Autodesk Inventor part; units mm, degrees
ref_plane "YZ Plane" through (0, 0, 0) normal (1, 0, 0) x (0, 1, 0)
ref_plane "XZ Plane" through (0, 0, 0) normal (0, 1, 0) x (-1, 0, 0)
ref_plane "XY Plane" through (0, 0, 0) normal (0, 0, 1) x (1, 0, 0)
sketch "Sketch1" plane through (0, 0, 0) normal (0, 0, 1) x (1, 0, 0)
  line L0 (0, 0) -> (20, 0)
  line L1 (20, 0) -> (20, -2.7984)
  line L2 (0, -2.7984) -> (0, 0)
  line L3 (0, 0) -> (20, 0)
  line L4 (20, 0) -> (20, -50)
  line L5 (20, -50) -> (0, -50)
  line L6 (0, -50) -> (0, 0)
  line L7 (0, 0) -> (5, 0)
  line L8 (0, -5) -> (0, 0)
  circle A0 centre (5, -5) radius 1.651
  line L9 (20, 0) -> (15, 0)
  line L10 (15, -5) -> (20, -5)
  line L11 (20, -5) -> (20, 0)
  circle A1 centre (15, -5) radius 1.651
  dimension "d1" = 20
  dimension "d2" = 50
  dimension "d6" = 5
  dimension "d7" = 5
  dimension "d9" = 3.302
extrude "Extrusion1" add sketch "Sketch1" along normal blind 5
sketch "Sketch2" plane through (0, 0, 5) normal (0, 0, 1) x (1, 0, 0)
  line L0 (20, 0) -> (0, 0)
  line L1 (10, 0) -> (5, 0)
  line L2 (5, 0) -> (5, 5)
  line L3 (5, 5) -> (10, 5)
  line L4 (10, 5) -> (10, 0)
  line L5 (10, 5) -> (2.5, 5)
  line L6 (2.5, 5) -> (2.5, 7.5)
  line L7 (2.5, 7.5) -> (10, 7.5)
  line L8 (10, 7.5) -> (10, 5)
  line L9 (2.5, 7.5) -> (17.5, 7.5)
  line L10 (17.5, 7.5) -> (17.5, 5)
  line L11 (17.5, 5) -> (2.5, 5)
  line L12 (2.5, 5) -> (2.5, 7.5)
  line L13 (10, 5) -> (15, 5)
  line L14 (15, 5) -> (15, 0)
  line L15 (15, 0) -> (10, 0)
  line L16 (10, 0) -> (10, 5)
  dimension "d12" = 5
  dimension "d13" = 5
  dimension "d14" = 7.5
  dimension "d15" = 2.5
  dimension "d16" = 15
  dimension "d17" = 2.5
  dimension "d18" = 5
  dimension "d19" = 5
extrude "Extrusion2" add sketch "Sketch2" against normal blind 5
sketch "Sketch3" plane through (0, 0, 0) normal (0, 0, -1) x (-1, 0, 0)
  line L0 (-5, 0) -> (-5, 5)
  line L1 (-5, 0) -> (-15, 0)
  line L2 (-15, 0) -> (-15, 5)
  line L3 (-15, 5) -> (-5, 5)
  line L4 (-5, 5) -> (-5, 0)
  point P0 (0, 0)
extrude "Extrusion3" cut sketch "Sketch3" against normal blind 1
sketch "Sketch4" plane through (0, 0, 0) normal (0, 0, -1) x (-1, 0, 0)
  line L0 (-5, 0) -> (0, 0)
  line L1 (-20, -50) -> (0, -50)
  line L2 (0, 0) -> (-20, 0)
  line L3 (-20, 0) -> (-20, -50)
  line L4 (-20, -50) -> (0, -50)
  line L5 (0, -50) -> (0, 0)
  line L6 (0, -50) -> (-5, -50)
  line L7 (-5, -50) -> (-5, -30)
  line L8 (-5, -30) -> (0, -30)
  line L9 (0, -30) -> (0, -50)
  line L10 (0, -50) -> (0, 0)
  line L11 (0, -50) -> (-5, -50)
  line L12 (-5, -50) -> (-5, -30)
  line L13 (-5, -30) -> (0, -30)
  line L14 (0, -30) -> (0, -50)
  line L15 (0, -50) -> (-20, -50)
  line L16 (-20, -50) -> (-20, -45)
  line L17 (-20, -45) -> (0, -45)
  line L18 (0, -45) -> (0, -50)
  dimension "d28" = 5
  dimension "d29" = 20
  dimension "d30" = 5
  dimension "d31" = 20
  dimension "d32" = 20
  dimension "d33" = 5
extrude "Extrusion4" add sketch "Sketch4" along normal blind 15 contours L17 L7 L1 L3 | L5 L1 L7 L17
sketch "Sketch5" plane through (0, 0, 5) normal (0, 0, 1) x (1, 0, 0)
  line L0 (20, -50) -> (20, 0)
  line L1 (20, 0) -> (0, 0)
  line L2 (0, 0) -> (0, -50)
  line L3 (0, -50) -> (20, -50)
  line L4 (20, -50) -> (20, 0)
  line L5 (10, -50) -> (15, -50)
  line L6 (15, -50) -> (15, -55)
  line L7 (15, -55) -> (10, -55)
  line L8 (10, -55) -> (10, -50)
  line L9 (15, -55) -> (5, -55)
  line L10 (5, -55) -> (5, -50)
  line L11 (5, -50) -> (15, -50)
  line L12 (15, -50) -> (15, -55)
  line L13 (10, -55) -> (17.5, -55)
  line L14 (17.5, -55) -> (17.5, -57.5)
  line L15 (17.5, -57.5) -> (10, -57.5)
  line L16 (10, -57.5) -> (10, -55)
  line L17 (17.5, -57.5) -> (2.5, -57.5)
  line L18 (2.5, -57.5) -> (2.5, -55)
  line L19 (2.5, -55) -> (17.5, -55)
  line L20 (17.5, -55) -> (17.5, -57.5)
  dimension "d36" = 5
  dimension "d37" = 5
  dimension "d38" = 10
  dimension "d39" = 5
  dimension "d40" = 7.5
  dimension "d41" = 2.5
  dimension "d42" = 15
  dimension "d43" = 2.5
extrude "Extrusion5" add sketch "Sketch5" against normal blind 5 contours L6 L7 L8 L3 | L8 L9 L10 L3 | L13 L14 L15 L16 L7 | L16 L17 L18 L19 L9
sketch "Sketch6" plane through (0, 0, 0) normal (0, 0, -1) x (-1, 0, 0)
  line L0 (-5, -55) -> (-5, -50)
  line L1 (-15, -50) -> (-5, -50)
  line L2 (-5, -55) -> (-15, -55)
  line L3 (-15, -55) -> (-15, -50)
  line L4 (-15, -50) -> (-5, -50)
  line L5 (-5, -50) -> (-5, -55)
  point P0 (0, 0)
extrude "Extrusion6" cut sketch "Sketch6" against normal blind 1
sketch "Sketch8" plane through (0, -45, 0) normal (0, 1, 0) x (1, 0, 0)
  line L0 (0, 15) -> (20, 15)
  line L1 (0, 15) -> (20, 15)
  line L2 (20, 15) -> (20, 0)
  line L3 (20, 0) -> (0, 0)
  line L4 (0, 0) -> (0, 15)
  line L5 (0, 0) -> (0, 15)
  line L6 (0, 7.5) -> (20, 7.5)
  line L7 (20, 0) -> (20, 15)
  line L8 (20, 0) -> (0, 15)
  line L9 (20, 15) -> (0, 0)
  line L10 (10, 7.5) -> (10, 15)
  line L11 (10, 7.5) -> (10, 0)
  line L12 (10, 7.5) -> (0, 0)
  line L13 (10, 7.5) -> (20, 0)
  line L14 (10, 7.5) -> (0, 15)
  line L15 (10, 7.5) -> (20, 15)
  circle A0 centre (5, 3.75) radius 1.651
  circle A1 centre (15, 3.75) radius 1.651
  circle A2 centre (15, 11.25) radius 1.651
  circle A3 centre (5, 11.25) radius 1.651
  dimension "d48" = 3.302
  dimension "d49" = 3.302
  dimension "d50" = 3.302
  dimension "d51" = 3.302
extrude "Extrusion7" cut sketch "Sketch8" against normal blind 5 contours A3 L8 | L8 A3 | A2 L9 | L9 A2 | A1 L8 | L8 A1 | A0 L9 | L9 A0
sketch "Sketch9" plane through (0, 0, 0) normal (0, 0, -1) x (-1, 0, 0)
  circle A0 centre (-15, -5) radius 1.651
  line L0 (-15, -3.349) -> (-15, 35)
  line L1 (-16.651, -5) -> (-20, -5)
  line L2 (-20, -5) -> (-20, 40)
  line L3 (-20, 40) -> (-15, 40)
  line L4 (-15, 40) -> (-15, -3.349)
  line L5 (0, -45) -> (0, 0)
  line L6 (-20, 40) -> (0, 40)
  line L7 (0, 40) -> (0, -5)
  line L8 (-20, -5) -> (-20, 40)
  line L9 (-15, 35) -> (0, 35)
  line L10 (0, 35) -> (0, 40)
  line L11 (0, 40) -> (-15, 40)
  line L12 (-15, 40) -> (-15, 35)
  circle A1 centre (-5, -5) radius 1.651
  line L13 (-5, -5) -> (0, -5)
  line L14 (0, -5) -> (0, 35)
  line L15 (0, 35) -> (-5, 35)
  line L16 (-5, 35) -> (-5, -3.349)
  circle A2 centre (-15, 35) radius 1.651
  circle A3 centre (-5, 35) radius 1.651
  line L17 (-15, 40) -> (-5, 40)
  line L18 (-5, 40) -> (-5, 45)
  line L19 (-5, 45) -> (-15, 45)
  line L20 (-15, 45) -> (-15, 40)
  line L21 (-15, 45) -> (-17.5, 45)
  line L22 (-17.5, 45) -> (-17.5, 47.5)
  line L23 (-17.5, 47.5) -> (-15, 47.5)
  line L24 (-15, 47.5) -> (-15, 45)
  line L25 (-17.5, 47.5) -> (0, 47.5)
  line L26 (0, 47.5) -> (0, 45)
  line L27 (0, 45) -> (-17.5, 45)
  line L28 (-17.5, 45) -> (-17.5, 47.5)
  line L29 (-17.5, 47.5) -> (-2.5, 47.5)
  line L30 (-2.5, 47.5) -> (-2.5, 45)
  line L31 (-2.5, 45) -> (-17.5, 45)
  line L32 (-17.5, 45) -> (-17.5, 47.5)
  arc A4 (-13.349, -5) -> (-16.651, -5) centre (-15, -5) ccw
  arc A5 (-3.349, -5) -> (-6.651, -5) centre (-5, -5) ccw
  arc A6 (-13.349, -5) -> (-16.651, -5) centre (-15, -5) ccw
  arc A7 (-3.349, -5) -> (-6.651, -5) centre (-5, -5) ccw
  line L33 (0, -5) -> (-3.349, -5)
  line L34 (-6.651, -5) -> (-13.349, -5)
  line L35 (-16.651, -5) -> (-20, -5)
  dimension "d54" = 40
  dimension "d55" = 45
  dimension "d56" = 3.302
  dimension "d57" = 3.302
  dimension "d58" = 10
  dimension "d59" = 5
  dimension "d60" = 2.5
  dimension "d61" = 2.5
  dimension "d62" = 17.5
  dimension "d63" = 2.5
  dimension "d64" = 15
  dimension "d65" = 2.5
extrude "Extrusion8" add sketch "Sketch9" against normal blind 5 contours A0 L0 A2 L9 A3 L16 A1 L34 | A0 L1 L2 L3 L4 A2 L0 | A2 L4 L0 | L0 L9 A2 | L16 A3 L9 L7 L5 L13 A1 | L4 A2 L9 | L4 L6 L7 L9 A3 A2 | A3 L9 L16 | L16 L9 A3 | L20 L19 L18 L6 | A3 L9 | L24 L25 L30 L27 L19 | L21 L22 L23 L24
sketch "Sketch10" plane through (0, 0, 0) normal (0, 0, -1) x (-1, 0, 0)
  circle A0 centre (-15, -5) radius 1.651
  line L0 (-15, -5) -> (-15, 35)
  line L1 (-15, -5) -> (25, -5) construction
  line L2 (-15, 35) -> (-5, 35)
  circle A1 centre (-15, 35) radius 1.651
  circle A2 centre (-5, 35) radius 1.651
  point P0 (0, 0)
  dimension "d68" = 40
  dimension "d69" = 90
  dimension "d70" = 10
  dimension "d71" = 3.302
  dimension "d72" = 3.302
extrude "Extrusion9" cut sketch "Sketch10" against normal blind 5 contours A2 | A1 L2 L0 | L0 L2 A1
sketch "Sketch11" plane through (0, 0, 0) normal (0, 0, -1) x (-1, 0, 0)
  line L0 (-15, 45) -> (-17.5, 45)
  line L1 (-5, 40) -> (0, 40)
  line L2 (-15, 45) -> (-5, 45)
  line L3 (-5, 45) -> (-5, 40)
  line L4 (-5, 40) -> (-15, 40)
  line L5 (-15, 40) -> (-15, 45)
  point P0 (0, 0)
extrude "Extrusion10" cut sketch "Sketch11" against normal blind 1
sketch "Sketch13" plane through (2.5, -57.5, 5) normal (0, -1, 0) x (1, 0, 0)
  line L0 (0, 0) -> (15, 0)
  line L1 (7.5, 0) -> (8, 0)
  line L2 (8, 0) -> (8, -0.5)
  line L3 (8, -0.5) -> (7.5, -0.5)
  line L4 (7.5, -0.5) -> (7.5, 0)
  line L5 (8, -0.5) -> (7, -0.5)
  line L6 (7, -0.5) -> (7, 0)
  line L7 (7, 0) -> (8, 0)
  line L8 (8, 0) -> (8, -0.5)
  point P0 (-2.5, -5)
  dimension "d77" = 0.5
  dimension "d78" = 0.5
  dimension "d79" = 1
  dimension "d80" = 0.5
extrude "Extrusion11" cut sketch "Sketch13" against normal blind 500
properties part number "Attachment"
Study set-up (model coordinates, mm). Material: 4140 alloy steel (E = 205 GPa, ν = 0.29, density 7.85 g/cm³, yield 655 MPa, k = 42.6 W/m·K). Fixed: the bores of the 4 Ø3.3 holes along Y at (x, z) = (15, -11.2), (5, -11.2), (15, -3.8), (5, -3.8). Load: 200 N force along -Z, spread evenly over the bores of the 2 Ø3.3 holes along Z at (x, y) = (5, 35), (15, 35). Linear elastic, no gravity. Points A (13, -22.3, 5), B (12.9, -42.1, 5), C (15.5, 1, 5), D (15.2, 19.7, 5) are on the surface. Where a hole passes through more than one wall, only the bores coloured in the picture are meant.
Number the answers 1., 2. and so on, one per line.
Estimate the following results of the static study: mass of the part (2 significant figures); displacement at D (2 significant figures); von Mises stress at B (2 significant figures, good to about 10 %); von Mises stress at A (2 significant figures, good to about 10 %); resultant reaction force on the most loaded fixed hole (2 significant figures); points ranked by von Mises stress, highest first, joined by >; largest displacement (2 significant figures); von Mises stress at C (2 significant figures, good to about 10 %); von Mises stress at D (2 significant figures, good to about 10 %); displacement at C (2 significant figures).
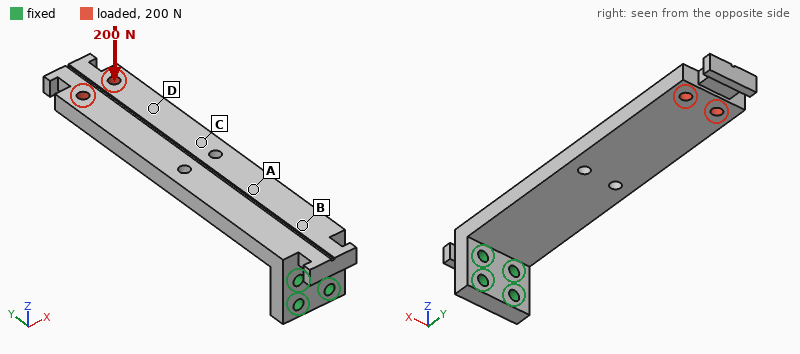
1. 85 g
2. 0.75 mm
3. 180 MPa
4. 140 MPa
5. 290 N
6. B > A > C > D
7. 1.3 mm
8. 78 MPa
9. 38 MPa
10. 0.45 mm
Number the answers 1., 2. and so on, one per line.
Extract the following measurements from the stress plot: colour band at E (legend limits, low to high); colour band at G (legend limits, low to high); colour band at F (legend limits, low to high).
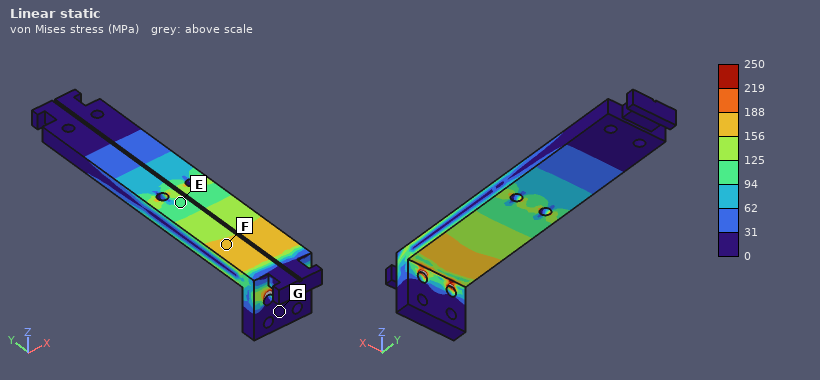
1. 94 to 125 MPa
2. 0 to 31 MPa
3. 156 to 188 MPa
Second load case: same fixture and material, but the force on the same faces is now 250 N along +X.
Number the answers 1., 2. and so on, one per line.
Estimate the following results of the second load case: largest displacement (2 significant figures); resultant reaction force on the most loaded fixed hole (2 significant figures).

1. 0.15 mm
2. 1.5 kN
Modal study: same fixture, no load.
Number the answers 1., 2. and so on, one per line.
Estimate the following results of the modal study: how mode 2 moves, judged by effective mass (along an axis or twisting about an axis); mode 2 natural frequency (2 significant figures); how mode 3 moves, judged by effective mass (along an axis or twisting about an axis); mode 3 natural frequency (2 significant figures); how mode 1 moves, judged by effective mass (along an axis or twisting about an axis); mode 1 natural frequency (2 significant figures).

1. along X
2. 1400 Hz
3. along Z
4. 2800 Hz
5. along Z
6. 460 Hz
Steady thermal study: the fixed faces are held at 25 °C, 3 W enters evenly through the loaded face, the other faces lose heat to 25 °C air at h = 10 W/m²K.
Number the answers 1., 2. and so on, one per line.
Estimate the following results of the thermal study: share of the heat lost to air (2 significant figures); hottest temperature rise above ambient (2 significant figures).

1. 40 %
2. 45 K
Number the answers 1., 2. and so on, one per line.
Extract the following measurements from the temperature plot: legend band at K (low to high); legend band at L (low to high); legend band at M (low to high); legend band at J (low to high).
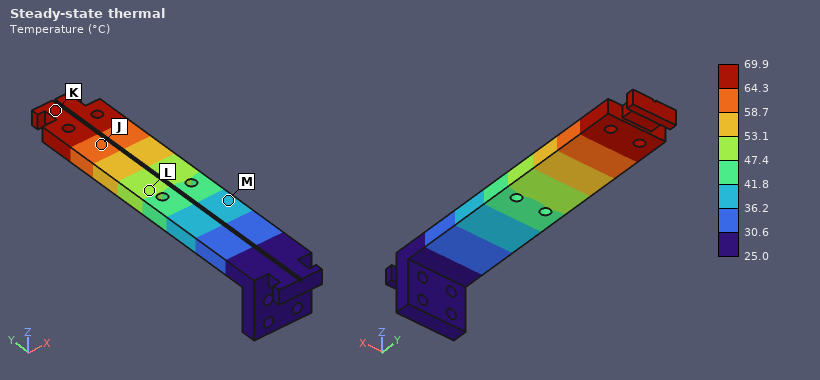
1. 64.3 to 69.9 °C
2. 47.4 to 53.1 °C
3. 36.2 to 41.8 °C
4. 58.7 to 64.3 °C
